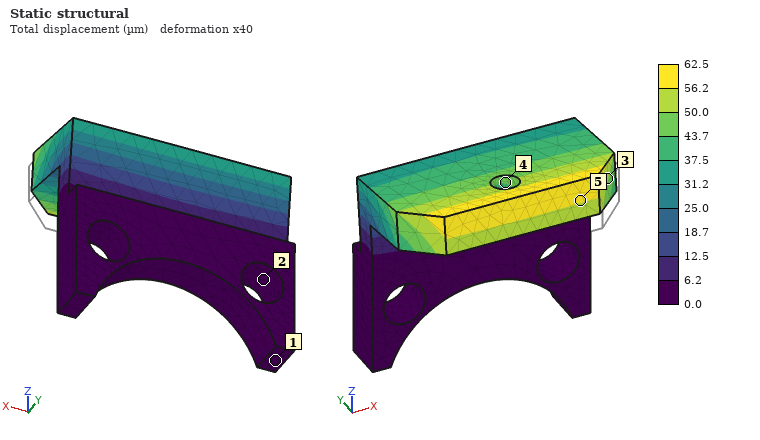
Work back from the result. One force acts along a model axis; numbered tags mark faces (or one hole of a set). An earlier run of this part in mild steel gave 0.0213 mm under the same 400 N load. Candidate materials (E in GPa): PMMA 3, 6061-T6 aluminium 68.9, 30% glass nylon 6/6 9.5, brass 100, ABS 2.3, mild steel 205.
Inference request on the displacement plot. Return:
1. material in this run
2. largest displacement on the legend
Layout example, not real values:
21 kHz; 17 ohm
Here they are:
6061-T6 aluminium; 62.5 µm
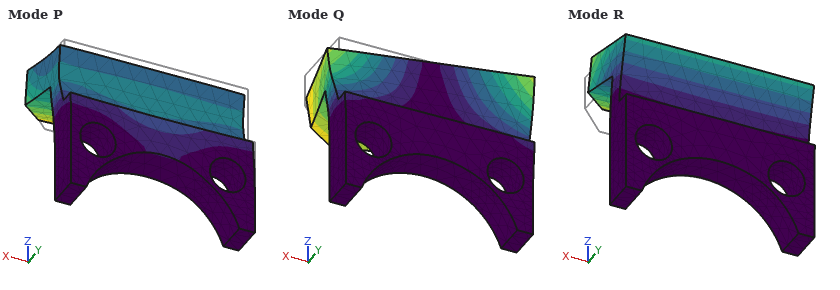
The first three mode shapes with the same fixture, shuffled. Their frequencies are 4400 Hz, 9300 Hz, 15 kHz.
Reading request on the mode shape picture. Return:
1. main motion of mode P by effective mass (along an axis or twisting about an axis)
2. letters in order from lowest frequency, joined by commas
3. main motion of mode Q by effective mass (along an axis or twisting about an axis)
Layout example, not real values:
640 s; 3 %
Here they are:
along Y; R, Q, P; along X
